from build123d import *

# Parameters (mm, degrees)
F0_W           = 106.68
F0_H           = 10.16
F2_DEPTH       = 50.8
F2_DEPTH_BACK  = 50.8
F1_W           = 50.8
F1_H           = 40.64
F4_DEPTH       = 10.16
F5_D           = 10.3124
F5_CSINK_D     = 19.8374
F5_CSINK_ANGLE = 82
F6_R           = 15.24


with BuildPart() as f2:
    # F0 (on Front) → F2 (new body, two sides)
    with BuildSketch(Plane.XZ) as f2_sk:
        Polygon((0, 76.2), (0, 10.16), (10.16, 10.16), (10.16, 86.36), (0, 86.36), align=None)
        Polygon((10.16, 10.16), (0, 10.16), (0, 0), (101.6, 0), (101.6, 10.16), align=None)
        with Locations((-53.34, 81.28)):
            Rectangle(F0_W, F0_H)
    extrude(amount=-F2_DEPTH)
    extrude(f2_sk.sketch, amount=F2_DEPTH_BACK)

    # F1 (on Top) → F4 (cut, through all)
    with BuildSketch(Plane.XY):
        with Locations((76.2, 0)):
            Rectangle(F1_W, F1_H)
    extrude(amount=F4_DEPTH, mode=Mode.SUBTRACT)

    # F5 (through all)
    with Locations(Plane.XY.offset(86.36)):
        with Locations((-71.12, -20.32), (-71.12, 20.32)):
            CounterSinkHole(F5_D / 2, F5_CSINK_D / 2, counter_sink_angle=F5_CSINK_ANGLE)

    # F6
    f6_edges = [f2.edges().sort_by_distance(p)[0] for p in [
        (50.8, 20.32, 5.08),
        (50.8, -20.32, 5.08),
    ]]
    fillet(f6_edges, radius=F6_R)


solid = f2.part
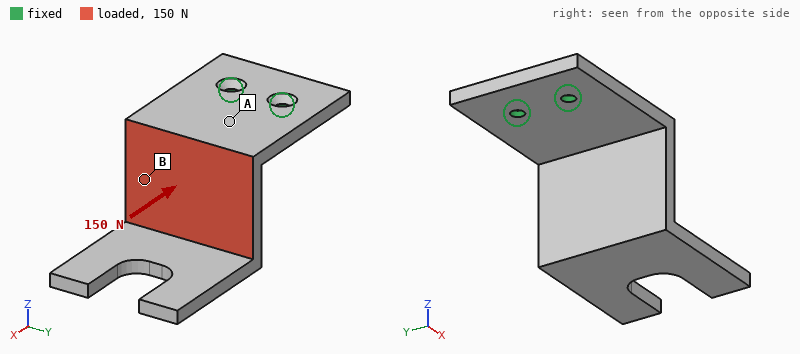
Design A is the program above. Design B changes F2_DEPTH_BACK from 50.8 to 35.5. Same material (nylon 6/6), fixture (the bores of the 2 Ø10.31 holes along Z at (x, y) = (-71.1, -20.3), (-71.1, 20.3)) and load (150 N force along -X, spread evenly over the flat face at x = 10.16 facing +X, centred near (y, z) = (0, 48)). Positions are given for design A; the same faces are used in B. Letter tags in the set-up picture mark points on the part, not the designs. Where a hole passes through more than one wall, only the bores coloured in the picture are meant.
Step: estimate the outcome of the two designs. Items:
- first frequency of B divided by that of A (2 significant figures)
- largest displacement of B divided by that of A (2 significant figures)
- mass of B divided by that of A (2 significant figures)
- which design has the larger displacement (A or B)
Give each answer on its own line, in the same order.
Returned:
1.0
1.2
0.84
B
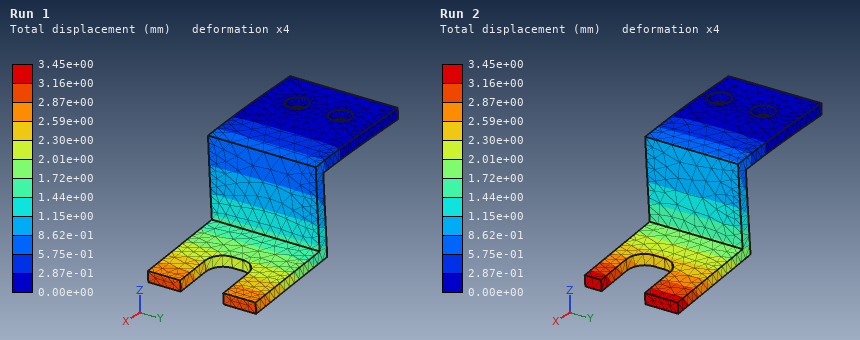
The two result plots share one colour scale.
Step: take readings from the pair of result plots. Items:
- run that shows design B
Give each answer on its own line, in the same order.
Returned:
Run 2
